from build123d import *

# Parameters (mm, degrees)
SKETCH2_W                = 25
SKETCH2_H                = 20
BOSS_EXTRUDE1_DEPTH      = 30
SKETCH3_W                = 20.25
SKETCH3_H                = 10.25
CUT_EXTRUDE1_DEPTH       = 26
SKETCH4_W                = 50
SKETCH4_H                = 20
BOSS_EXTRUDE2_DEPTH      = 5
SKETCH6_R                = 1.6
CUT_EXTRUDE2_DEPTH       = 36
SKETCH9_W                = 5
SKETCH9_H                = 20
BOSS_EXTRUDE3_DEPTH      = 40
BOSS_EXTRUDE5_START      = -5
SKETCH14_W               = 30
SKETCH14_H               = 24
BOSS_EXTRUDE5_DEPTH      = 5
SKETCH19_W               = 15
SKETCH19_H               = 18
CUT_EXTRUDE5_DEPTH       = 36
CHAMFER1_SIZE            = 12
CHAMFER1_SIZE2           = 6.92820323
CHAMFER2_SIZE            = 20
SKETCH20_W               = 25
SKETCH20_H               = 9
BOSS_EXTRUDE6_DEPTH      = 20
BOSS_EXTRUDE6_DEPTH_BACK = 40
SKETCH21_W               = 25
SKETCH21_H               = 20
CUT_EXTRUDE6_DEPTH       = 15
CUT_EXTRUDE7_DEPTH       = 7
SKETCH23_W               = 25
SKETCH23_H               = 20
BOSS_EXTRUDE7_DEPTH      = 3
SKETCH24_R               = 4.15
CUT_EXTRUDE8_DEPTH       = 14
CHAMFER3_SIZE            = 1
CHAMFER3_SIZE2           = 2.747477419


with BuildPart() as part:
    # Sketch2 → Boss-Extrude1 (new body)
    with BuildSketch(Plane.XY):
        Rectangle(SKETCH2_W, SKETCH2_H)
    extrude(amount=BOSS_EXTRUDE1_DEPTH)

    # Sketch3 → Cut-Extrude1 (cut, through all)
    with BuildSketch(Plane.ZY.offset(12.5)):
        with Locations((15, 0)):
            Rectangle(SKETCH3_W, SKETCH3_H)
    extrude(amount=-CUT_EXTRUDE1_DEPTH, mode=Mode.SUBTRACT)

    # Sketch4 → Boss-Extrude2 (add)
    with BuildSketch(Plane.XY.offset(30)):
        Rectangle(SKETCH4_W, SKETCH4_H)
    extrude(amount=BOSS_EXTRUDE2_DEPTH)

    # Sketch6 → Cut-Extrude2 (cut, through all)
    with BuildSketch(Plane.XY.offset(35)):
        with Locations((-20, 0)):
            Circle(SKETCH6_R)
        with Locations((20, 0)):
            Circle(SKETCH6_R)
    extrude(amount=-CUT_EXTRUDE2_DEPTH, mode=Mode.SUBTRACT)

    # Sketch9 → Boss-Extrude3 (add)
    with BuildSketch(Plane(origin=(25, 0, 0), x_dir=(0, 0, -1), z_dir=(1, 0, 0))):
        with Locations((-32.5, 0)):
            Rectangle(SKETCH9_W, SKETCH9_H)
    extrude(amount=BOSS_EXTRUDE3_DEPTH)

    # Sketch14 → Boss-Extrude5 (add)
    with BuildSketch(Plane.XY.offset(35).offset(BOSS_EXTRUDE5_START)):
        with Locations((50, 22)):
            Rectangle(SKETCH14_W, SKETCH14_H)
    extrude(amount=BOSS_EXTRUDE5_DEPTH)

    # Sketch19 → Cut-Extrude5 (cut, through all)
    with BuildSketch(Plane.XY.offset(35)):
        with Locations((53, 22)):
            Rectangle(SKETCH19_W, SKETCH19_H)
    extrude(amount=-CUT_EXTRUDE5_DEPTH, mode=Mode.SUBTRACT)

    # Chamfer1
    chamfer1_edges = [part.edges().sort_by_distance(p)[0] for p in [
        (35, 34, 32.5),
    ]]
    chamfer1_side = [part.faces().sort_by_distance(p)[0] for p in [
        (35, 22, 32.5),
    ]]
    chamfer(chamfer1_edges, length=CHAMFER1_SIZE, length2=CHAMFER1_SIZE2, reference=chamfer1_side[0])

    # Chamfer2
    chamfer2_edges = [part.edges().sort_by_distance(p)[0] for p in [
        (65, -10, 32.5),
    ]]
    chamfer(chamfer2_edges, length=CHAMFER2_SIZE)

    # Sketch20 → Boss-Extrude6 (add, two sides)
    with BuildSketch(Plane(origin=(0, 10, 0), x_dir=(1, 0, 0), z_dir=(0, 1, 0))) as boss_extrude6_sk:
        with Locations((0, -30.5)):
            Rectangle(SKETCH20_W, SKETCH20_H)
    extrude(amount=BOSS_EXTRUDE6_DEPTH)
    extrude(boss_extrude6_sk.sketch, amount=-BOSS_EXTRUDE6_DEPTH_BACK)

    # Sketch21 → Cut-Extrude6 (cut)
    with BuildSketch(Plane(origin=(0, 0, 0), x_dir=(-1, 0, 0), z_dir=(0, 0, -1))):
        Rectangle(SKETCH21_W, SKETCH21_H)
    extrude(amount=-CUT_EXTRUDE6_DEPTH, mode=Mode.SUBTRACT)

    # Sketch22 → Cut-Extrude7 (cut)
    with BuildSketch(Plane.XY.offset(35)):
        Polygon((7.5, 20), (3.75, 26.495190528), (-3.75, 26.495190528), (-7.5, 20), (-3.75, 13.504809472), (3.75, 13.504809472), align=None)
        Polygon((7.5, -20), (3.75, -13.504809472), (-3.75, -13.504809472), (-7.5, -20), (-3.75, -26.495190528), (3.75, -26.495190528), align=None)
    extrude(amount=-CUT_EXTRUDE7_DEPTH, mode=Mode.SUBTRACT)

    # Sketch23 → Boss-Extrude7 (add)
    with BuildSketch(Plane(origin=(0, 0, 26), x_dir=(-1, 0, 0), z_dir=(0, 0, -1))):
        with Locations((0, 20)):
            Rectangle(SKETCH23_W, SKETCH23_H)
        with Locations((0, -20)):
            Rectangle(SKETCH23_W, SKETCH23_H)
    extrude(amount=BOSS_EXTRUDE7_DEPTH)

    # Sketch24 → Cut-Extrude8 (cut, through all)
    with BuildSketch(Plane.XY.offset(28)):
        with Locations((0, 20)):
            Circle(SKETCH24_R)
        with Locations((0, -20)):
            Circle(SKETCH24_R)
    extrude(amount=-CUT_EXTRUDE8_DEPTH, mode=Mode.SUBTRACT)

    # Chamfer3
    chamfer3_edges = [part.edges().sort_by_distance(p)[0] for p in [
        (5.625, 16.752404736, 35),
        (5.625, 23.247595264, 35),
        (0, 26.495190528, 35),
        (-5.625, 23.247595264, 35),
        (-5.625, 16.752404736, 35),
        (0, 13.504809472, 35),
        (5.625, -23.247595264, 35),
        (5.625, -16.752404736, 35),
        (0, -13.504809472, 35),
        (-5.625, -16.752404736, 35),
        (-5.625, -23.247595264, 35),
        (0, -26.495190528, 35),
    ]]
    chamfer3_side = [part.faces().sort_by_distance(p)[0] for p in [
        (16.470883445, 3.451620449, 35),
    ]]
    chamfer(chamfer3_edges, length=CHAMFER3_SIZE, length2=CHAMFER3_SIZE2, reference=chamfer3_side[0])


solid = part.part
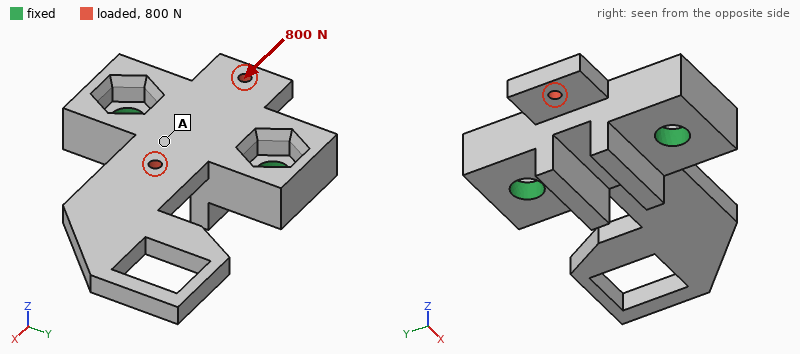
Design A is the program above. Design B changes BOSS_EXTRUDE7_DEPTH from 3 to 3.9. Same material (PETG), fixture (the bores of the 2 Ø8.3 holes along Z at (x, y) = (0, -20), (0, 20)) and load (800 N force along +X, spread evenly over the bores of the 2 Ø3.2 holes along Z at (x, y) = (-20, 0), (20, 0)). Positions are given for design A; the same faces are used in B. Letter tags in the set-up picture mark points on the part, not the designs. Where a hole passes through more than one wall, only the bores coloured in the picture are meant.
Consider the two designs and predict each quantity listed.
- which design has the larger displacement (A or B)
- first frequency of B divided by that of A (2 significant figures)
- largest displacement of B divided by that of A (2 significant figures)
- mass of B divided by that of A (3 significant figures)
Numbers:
A
1.0
0.87
1.03
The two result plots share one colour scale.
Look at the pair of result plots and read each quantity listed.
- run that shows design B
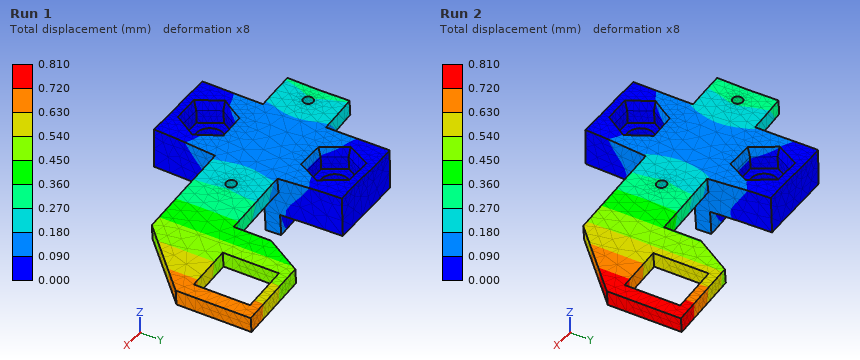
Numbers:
Run 1
